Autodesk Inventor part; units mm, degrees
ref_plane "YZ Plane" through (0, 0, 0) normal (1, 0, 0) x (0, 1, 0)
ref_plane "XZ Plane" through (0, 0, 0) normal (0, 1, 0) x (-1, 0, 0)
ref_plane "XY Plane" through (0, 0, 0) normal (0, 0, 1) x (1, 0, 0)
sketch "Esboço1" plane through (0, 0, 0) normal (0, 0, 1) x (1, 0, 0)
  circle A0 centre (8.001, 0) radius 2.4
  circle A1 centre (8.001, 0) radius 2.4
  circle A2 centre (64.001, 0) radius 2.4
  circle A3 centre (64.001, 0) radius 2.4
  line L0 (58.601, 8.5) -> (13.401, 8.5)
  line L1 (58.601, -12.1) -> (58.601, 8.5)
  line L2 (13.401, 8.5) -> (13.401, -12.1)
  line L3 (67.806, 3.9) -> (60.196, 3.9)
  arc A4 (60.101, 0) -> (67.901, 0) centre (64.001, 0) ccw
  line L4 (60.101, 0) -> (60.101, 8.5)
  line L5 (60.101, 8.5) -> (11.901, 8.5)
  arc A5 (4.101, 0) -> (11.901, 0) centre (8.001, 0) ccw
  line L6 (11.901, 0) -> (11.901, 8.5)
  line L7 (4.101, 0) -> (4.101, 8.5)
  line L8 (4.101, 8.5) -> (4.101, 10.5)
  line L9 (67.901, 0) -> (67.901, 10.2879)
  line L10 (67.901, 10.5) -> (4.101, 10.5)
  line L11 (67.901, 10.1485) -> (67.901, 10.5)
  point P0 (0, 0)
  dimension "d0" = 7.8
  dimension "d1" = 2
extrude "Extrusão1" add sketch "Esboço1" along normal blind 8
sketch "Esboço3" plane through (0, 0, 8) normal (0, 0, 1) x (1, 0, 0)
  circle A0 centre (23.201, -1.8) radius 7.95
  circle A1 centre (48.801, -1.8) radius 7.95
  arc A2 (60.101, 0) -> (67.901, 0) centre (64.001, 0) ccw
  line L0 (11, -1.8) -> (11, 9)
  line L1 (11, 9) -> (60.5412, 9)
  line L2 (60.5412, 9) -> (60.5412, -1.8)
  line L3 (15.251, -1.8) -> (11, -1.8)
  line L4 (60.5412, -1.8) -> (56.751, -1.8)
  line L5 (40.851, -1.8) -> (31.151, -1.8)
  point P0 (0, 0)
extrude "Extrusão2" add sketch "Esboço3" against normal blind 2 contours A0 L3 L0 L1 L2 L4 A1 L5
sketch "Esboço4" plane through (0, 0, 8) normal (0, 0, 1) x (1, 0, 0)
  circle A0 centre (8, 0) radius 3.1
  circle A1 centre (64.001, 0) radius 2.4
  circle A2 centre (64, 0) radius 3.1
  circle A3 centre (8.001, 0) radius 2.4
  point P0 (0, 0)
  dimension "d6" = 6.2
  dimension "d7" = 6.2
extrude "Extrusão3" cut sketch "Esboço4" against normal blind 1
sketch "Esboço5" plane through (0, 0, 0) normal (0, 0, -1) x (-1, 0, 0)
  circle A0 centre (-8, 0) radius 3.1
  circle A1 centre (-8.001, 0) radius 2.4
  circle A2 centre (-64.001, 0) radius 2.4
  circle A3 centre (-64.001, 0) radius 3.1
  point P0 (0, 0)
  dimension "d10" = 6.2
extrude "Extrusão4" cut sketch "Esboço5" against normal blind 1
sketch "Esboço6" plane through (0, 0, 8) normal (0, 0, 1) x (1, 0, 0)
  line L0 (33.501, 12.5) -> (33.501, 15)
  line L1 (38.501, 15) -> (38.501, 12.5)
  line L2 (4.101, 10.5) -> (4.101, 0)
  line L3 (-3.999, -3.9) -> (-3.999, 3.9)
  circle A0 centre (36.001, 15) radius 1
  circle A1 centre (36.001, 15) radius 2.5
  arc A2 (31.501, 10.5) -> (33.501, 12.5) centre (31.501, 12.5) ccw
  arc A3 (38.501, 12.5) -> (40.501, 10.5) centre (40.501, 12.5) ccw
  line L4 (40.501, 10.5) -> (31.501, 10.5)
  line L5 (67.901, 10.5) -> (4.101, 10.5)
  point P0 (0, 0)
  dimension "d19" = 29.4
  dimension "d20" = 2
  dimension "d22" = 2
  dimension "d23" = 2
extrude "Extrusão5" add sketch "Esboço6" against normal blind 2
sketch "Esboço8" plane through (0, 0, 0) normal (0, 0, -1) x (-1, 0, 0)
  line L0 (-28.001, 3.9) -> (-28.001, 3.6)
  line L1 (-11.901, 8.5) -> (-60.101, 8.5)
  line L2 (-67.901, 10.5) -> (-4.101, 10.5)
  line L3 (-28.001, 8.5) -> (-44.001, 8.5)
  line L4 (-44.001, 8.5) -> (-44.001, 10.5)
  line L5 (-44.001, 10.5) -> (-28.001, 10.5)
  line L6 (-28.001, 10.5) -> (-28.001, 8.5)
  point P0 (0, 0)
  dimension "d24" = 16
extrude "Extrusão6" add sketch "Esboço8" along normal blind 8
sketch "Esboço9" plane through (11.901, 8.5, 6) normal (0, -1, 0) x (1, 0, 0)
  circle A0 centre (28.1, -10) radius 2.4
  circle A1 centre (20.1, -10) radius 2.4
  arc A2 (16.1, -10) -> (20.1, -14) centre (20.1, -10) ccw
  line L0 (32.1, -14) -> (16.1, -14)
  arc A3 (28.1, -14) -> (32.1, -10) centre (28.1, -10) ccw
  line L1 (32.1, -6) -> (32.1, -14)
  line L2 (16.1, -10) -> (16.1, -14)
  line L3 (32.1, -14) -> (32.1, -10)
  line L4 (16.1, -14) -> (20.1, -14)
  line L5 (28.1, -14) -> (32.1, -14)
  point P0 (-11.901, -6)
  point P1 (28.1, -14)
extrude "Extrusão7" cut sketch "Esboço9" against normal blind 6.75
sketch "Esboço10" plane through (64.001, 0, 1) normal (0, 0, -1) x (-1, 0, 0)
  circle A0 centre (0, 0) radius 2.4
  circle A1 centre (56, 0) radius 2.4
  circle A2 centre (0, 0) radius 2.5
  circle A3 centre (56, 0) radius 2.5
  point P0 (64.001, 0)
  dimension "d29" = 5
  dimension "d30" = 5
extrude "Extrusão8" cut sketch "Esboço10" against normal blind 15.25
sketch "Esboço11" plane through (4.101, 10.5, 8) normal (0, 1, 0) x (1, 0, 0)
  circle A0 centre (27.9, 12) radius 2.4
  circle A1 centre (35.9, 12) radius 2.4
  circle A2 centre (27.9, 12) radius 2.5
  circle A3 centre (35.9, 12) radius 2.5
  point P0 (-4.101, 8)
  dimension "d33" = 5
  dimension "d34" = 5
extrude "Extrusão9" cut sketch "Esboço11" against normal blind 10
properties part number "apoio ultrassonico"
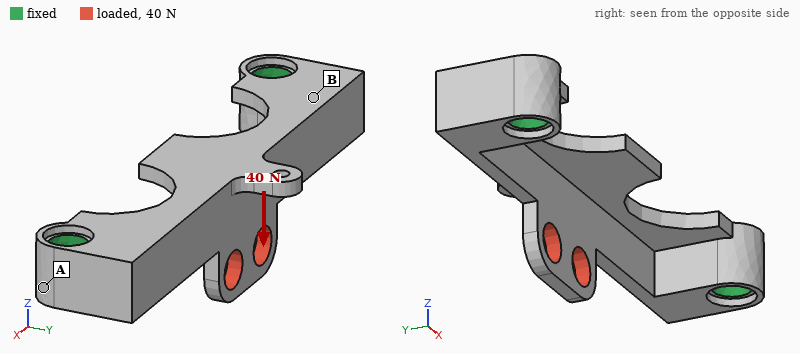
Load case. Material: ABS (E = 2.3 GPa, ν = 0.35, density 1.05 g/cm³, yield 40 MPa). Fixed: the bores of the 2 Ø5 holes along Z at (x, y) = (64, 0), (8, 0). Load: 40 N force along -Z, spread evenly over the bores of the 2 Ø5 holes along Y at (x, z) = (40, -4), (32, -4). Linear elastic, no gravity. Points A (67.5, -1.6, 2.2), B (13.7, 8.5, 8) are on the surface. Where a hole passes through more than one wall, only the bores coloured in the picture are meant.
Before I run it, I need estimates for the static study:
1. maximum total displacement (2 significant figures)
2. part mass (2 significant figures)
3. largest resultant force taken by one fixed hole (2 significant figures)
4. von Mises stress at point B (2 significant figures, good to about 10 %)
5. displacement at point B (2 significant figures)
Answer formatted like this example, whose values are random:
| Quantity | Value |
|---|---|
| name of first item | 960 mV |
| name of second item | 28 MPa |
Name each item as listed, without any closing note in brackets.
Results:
| Quantity | Value |
|---|---|
| maximum total displacement | 0.20 mm |
| part mass | 3.1 g |
| largest resultant force taken by one fixed hole | 20 N |
| von Mises stress at point B | 3.4 MPa |
| displacement at point B | 0.040 mm |
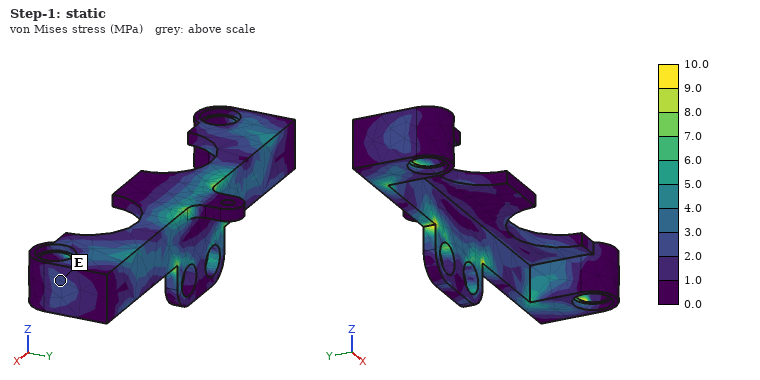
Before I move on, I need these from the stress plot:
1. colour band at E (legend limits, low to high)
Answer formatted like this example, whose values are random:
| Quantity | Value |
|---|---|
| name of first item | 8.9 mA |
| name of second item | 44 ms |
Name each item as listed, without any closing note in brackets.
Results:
| Quantity | Value |
|---|---|
| colour band at E | 2.0 to 3.0 MPa |
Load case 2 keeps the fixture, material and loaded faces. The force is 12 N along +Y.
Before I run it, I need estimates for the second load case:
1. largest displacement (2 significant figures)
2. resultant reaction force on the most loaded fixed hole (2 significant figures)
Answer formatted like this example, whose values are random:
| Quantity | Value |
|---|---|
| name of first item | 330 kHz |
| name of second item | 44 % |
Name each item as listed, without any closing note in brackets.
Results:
| Quantity | Value |
|---|---|
| largest displacement | 0.79 mm |
| resultant reaction force on the most loaded fixed hole | 8.4 N |
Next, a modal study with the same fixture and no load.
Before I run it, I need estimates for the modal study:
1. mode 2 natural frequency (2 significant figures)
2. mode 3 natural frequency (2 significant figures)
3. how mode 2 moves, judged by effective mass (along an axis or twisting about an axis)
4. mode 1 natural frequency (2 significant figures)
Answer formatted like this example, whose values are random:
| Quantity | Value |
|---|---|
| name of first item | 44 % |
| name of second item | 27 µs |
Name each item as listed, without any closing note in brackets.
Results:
| Quantity | Value |
|---|---|
| mode 2 natural frequency | 2200 Hz |
| mode 3 natural frequency | 3600 Hz |
| how mode 2 moves, judged by effective mass | along Z |
| mode 1 natural frequency | 1400 Hz |
